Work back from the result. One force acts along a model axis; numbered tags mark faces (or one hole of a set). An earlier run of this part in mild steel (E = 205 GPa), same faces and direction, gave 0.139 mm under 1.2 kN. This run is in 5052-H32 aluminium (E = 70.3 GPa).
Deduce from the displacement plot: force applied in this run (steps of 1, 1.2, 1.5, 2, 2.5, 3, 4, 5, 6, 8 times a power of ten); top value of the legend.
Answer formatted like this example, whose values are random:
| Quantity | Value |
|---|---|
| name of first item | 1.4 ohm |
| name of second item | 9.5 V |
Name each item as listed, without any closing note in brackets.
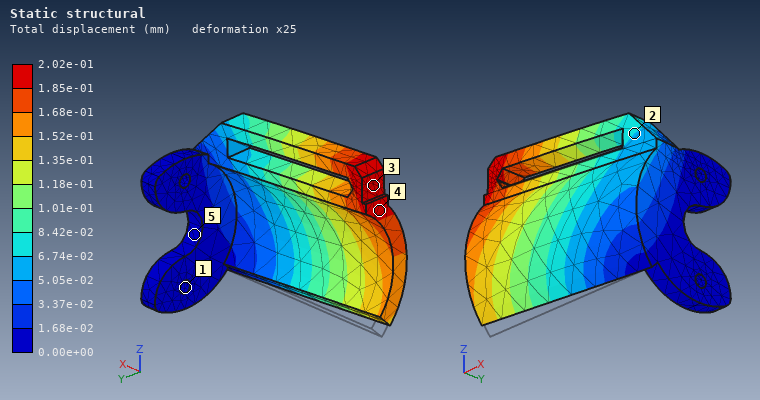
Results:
| Quantity | Value |
|---|---|
| force applied in this run | 600 N |
| top value of the legend | 2.02e-01 mm |
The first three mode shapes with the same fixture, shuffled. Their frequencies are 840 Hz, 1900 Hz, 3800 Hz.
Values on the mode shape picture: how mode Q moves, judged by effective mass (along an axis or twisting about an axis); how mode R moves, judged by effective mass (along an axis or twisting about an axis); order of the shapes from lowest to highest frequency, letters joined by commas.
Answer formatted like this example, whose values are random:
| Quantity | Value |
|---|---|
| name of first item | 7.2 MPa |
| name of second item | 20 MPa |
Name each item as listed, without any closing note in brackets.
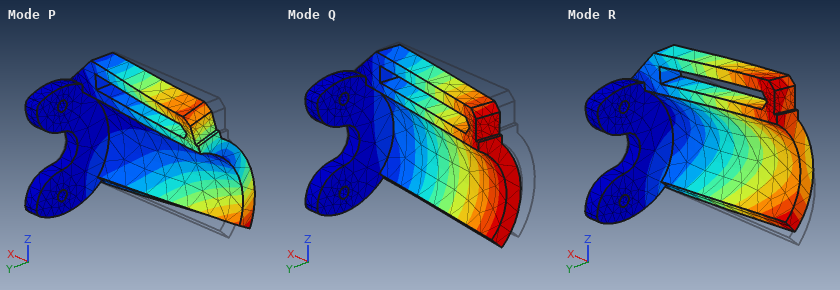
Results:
| Quantity | Value |
|---|---|
| how mode Q moves, judged by effective mass | along Y |
| how mode R moves, judged by effective mass | along Z |
| order of the shapes from lowest to highest frequency, letters joined by commas | Q, R, P |
